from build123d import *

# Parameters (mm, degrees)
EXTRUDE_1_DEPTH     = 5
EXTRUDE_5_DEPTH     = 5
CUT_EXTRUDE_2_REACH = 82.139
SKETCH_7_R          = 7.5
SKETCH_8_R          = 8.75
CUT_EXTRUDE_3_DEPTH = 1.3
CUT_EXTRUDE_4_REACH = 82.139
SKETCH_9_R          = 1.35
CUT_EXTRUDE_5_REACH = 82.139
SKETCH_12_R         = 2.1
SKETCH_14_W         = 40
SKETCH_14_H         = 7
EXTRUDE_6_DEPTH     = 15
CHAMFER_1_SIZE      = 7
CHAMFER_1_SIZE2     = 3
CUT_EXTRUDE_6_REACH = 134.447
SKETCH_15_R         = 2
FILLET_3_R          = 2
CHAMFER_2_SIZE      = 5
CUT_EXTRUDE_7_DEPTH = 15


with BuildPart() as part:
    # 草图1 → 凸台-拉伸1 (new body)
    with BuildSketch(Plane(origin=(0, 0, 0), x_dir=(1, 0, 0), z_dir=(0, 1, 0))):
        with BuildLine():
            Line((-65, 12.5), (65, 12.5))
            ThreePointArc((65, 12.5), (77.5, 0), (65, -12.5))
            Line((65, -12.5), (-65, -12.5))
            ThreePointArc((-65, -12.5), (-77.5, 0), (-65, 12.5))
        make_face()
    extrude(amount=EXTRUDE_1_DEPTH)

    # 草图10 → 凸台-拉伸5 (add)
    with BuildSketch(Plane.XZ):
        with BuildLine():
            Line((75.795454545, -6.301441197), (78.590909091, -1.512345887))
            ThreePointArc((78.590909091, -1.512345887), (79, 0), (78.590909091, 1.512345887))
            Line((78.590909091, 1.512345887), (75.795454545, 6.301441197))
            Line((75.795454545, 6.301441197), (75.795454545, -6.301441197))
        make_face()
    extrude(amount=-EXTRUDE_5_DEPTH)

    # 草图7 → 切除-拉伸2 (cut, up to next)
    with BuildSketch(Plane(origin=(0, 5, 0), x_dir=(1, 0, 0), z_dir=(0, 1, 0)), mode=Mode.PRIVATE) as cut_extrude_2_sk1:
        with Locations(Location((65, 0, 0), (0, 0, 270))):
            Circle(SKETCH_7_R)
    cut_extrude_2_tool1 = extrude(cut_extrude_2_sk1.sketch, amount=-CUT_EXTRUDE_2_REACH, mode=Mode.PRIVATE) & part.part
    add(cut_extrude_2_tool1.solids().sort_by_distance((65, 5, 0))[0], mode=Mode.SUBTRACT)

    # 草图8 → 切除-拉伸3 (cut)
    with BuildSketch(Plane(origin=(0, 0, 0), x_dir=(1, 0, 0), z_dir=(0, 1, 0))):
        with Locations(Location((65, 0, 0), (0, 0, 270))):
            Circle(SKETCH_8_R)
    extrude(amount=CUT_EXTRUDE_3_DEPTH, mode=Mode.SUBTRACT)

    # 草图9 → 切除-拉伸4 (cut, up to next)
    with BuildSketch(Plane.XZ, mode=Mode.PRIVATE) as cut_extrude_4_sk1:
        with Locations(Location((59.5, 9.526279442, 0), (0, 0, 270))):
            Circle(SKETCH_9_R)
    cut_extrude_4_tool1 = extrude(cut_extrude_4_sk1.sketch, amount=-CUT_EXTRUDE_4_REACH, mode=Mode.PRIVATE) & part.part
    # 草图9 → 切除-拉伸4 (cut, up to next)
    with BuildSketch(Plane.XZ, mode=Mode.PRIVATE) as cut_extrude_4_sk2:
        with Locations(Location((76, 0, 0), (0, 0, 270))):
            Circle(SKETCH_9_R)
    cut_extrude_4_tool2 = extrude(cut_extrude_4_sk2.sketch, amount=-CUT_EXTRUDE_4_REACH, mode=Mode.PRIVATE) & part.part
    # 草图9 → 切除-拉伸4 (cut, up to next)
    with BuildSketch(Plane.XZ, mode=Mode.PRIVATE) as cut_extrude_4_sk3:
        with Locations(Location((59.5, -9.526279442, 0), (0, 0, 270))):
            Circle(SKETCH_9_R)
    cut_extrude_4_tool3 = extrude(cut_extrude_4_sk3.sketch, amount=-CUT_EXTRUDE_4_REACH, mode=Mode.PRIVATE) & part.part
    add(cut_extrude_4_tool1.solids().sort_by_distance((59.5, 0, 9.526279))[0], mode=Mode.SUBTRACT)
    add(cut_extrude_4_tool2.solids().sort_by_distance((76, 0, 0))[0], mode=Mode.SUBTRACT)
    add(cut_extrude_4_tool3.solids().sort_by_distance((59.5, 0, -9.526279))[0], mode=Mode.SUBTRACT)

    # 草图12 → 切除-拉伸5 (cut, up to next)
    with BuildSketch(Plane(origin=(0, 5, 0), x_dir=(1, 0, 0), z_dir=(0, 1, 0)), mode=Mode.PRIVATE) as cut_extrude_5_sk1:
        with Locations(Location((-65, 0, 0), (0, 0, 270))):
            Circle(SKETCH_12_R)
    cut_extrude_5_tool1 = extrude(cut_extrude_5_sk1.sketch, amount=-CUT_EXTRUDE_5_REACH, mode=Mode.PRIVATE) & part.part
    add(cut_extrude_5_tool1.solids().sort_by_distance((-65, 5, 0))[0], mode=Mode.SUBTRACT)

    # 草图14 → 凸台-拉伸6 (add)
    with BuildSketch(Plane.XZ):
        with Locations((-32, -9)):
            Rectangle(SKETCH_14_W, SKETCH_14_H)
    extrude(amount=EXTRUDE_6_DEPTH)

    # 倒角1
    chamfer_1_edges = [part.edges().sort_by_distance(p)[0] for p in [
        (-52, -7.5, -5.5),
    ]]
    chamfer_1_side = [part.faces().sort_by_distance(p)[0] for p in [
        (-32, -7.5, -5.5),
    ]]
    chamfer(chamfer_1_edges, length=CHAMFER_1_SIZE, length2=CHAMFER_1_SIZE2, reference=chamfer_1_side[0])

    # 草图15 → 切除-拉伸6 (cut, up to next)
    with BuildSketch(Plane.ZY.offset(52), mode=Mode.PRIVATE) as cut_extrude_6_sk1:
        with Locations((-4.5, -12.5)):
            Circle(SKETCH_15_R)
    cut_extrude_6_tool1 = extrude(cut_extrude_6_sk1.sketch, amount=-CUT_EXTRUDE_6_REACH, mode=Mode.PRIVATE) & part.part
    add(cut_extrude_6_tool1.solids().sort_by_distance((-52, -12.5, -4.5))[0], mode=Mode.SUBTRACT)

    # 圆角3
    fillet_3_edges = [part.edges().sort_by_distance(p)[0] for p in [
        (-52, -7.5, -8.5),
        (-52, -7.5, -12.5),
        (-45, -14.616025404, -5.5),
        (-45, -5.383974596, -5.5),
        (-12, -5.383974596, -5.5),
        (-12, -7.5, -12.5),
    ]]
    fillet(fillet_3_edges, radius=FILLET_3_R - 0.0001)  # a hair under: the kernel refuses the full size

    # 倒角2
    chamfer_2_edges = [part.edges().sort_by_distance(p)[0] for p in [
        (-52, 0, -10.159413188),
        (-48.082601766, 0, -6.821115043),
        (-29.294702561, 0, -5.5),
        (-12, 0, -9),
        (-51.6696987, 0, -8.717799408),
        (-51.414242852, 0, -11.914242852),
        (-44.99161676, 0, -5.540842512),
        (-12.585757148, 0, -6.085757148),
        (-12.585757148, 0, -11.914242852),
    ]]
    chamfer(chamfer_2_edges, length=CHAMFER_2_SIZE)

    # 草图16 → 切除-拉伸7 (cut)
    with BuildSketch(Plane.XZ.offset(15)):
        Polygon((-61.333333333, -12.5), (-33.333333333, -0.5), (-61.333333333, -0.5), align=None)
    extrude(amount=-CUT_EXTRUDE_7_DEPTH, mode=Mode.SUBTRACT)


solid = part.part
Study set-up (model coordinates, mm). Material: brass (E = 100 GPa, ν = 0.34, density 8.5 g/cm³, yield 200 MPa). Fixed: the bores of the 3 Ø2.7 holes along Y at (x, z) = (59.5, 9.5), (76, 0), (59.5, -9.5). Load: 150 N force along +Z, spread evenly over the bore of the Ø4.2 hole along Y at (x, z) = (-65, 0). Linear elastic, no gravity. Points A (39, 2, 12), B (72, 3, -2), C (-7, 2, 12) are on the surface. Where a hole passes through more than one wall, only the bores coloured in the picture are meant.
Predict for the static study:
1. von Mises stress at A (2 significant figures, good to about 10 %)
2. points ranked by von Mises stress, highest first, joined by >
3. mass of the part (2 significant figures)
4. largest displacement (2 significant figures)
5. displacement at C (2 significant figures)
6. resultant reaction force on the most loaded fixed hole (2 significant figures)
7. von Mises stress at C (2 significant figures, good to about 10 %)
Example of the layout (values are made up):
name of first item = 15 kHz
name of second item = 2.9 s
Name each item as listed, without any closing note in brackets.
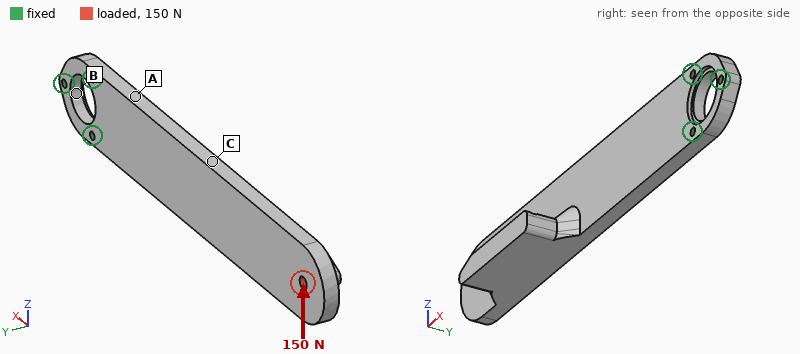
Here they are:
von Mises stress at A = 30 MPa
points ranked by von Mises stress, highest first, joined by > = A > C > B
mass of the part = 190 g
largest displacement = 0.17 mm
displacement at C = 0.058 mm
resultant reaction force on the most loaded fixed hole = 960 N
von Mises stress at C = 16 MPa
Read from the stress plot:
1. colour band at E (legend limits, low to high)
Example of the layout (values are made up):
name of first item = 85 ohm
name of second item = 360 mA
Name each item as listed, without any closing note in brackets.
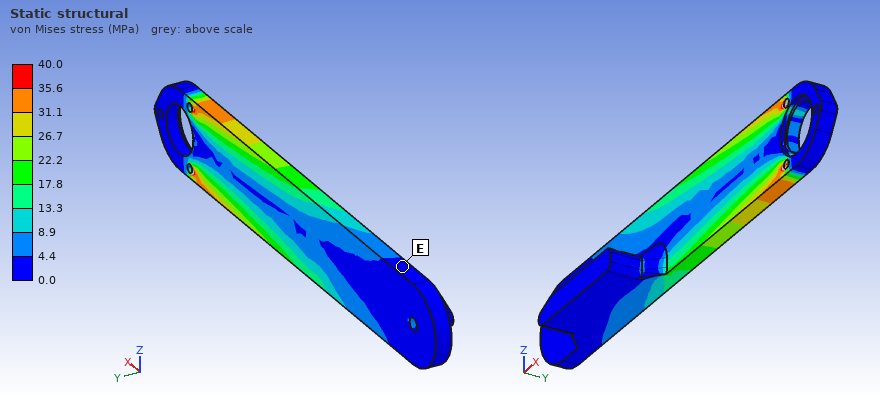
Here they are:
colour band at E = 0.0 to 4.4 MPa
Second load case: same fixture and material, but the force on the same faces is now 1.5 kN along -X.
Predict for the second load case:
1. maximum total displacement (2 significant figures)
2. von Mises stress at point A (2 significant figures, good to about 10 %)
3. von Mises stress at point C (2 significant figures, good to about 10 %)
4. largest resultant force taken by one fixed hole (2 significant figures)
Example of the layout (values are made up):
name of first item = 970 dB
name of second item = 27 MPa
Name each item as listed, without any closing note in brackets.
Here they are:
maximum total displacement = 24 µm
von Mises stress at point A = 12 MPa
von Mises stress at point C = 12 MPa
largest resultant force taken by one fixed hole = 780 N
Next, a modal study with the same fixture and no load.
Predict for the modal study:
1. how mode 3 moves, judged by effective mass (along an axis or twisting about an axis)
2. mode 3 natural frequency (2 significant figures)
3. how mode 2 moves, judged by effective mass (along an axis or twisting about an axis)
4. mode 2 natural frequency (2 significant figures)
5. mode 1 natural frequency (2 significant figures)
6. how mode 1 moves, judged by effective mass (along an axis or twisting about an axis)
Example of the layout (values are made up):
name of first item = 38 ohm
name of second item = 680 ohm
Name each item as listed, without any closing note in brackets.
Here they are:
how mode 3 moves, judged by effective mass = along Y
mode 3 natural frequency = 1000 Hz
how mode 2 moves, judged by effective mass = along Z
mode 2 natural frequency = 640 Hz
mode 1 natural frequency = 130 Hz
how mode 1 moves, judged by effective mass = along Y
